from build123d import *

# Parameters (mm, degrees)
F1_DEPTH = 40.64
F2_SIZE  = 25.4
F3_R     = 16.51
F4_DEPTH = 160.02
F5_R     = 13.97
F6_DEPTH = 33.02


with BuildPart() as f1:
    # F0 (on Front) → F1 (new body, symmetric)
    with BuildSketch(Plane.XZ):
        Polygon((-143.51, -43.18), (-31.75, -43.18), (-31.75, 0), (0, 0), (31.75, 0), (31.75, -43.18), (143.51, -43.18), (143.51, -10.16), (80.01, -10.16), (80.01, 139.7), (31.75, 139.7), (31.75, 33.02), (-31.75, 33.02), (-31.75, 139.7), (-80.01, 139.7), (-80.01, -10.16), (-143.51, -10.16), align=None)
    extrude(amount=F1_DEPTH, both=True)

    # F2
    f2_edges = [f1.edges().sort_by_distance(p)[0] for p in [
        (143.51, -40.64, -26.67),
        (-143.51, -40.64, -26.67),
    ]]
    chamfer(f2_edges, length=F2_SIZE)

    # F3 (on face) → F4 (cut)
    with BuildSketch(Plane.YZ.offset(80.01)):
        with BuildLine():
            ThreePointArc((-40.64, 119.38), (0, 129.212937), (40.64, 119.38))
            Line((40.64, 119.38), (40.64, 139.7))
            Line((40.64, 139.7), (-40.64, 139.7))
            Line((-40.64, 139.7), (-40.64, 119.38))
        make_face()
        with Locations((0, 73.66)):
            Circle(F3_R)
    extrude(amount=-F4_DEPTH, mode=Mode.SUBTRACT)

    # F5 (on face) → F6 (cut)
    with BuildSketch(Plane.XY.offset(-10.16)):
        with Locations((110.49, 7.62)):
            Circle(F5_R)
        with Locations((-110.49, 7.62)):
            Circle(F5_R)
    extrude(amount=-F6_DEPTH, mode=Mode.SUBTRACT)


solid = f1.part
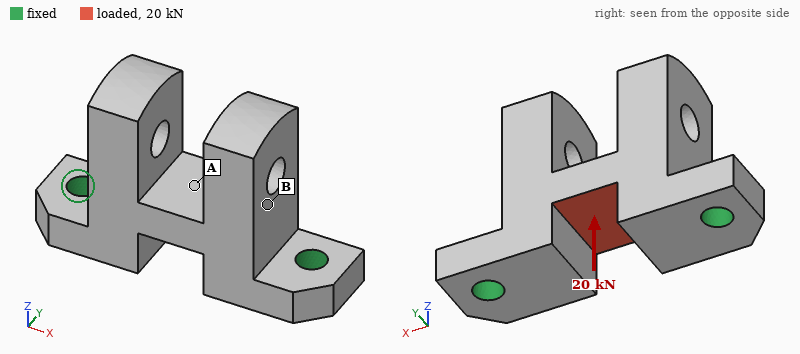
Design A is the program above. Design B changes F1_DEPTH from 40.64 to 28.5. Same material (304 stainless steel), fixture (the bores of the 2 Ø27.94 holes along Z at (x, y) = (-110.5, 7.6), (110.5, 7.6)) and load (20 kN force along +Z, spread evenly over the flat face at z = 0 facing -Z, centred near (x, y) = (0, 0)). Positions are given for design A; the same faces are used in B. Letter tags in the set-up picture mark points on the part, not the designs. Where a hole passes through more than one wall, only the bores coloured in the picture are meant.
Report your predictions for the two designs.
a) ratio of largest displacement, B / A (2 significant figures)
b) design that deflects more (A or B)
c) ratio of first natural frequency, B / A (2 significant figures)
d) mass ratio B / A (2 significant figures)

1.3
B
0.92
0.68
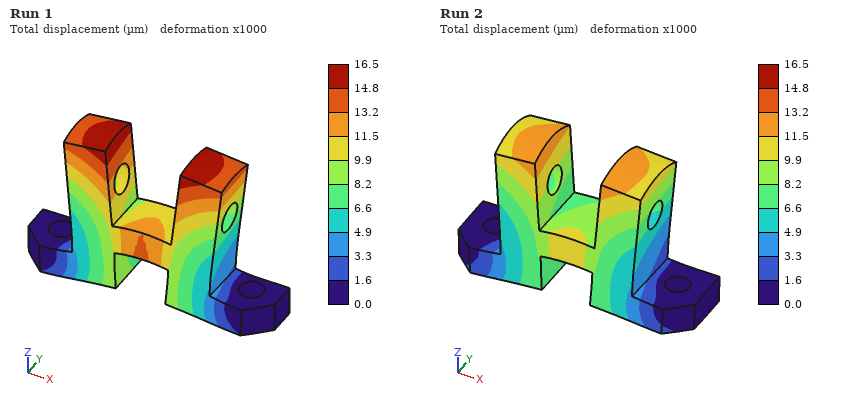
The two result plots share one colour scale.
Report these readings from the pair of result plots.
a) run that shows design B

Run 1
